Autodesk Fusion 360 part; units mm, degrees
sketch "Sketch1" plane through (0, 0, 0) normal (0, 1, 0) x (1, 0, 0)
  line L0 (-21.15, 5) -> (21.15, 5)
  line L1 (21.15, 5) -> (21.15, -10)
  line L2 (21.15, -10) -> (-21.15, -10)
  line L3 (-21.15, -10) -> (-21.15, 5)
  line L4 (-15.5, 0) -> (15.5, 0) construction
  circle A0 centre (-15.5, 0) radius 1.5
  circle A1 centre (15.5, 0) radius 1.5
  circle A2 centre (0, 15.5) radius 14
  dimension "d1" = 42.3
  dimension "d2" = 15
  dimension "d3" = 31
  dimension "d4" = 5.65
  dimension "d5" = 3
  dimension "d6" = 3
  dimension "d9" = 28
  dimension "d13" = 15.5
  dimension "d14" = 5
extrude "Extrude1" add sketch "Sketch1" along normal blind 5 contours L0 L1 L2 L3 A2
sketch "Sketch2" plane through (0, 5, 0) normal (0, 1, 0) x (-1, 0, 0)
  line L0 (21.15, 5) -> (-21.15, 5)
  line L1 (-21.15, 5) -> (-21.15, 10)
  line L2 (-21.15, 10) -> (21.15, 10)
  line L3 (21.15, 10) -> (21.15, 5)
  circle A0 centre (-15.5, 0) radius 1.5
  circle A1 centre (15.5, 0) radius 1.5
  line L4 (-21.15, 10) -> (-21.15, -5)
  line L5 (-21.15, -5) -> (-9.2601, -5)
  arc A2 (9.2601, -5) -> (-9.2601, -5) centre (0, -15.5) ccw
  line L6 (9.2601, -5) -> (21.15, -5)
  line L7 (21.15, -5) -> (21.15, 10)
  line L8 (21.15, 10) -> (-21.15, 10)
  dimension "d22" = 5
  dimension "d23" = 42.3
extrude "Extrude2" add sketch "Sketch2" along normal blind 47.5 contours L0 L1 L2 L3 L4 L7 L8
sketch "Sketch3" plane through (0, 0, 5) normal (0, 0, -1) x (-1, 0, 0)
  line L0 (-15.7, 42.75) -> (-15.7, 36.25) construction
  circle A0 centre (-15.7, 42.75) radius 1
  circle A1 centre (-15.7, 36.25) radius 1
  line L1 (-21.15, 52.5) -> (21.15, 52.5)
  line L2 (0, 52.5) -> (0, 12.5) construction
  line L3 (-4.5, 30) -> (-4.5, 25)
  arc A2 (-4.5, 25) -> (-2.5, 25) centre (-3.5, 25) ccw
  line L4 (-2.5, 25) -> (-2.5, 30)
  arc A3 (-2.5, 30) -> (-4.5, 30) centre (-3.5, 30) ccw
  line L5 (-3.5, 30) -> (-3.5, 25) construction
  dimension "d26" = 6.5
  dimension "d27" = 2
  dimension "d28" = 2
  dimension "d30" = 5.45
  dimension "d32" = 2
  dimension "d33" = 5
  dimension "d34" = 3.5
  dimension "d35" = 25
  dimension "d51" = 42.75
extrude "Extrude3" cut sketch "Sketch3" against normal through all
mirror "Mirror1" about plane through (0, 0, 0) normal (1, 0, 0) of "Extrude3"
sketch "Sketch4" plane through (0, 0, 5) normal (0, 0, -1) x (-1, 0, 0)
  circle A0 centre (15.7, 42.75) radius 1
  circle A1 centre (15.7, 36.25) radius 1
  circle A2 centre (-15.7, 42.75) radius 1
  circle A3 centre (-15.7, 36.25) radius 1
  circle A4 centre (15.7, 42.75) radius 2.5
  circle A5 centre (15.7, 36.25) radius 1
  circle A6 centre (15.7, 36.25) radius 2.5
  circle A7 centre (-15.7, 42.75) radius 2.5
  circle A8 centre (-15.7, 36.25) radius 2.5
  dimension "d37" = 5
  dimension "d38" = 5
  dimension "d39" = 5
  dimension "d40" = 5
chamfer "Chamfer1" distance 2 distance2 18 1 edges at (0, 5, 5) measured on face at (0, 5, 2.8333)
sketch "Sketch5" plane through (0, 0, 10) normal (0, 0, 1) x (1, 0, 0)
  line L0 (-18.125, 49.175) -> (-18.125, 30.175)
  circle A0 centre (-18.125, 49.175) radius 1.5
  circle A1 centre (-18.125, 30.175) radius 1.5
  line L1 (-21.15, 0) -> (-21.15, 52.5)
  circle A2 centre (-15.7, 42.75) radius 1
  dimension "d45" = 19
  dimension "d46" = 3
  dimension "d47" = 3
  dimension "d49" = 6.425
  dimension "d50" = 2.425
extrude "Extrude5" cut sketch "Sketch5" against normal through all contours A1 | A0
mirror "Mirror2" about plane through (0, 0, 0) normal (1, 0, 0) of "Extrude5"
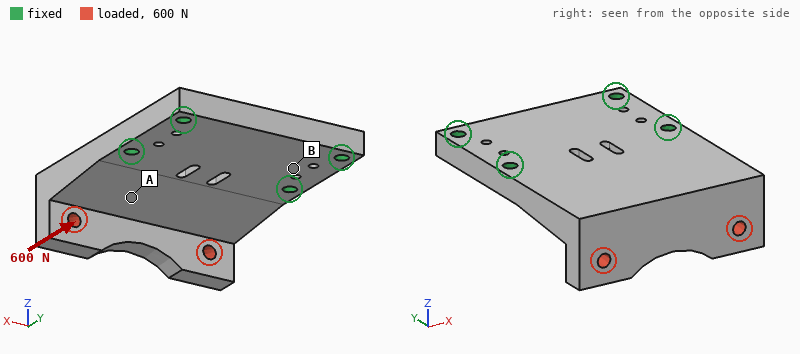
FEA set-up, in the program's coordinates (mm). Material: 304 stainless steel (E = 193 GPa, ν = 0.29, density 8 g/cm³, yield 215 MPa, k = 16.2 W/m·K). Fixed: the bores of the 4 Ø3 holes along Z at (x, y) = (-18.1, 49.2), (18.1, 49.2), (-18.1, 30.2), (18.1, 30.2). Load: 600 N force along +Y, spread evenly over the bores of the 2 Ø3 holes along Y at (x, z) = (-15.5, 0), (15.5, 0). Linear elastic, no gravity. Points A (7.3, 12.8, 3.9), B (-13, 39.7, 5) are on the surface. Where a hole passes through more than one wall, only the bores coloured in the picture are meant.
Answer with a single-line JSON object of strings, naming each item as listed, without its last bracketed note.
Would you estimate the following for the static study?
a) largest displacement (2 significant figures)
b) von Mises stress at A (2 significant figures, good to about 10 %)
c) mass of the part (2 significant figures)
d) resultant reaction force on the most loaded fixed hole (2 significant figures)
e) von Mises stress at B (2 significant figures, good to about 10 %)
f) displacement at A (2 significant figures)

{"largest displacement": "28 µm", "von Mises stress at A": "16 MPa", "mass of the part": "110 g", "resultant reaction force on the most loaded fixed hole": "250 N", "von Mises stress at B": "4.5 MPa", "displacement at A": "11 µm"}
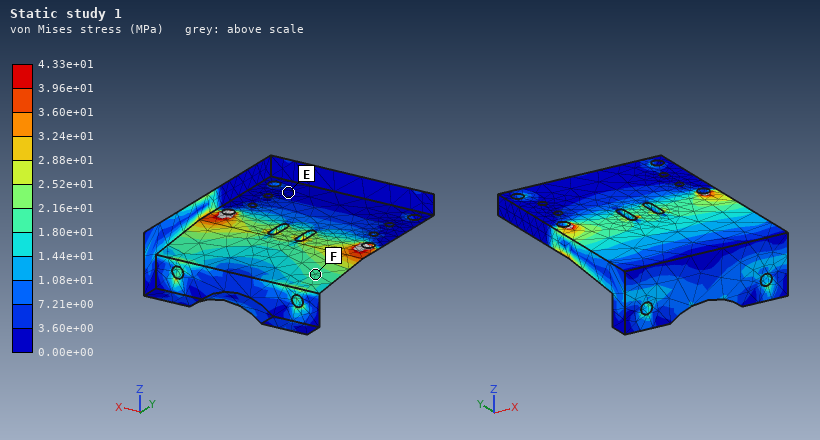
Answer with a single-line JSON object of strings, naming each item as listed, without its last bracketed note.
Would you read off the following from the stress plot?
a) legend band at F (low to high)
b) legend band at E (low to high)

{"legend band at F": "1.80e+01 to 2.16e+01 MPa", "legend band at E": "0.00e+00 to 3.60e+00 MPa"}
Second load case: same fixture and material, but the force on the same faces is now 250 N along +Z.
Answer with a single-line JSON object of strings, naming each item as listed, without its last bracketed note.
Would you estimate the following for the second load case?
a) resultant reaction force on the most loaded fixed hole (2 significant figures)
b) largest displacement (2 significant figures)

{"resultant reaction force on the most loaded fixed hole": "200 N", "largest displacement": "31 µm"}
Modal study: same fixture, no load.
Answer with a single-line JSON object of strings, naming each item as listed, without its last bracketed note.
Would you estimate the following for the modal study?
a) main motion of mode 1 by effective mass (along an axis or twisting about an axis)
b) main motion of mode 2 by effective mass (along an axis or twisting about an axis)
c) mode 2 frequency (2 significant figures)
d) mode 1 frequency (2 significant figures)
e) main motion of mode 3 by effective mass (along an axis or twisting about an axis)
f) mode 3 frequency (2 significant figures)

{"main motion of mode 1 by effective mass": "along Z", "main motion of mode 2 by effective mass": "twisting about Y", "mode 2 frequency": "6600 Hz", "mode 1 frequency": "2600 Hz", "main motion of mode 3 by effective mass": "along X", "mode 3 frequency": "14 kHz"}
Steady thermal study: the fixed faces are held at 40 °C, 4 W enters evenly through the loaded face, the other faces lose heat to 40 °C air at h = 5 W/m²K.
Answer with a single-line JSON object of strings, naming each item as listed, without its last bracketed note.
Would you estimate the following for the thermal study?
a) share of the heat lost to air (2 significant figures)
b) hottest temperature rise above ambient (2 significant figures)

{"share of the heat lost to air": "12 %", "hottest temperature rise above ambient": "43 K"}
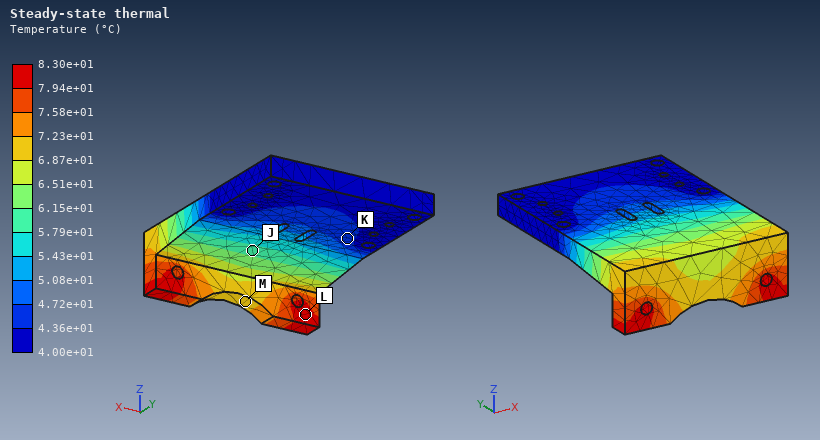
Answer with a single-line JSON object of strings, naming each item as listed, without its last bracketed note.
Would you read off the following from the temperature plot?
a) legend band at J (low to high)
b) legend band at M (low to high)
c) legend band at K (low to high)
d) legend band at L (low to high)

{"legend band at J": "5.79e+01 to 6.15e+01 °C", "legend band at M": "6.87e+01 to 7.23e+01 °C", "legend band at K": "4.36e+01 to 4.72e+01 °C", "legend band at L": "7.94e+01 to 8.30e+01 °C"}
